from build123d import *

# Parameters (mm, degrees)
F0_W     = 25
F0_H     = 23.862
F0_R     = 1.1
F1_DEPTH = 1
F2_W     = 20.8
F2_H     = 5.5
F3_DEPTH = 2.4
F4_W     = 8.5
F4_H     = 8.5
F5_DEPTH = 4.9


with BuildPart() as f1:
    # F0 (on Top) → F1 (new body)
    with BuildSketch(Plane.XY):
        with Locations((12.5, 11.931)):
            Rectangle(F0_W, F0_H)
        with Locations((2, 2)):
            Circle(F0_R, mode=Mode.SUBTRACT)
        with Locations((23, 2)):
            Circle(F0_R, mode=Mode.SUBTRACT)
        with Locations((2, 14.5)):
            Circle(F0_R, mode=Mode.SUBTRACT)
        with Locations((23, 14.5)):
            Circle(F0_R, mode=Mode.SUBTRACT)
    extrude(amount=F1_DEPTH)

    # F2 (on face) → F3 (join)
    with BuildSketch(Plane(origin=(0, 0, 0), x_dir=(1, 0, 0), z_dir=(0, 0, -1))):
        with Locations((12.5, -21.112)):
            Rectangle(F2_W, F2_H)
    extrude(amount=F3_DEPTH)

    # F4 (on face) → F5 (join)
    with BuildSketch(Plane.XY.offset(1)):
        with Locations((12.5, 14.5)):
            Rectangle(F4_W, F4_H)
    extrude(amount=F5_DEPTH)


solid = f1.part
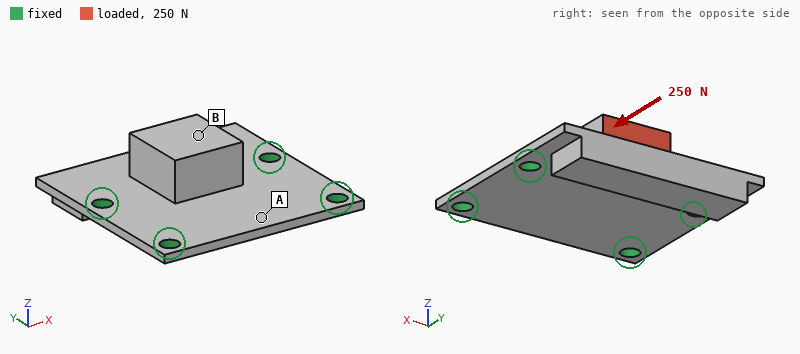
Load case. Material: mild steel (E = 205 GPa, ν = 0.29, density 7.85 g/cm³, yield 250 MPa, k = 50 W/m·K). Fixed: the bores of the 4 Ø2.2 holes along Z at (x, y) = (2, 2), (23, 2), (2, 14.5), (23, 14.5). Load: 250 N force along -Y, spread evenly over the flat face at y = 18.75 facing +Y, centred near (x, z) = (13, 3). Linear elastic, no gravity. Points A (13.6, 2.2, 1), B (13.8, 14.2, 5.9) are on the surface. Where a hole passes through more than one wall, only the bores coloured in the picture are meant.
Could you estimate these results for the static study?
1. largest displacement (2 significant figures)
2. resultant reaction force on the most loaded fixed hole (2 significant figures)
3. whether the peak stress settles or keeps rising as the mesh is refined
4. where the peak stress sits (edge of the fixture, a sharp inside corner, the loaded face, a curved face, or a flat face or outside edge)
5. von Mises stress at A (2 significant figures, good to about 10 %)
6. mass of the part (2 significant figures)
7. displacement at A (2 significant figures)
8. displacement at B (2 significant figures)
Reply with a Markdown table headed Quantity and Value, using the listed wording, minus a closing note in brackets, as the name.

| Quantity | Value |
|---|---|
| largest displacement | 17 µm |
| resultant reaction force on the most loaded fixed hole | 92 N |
| whether the peak stress settles or keeps rising as the mesh is refined | keeps rising |
| where the peak stress sits | edge of the fixture |
| von Mises stress at A | 23 MPa |
| mass of the part | 9.5 g |
| displacement at A | 6.6 µm |
| displacement at B | 10 µm |
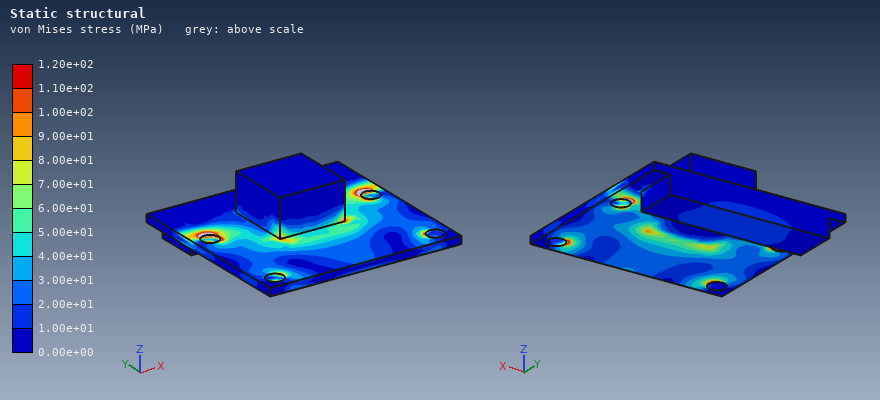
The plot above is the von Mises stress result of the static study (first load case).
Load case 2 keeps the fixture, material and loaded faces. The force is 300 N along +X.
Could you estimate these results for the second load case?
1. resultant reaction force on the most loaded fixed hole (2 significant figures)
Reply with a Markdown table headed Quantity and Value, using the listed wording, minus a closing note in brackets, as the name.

| Quantity | Value |
|---|---|
| resultant reaction force on the most loaded fixed hole | 150 N |
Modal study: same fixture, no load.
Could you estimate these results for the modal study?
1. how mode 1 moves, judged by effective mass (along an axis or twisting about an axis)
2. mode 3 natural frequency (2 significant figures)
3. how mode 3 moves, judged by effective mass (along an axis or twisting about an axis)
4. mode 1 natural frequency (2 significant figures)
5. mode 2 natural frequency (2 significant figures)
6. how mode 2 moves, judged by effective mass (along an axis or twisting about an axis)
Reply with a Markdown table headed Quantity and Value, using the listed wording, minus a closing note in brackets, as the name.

| Quantity | Value |
|---|---|
| how mode 1 moves, judged by effective mass | along Z |
| mode 3 natural frequency | 18 kHz |
| how mode 3 moves, judged by effective mass | twisting about Y |
| mode 1 natural frequency | 6200 Hz |
| mode 2 natural frequency | 11 kHz |
| how mode 2 moves, judged by effective mass | along Z |
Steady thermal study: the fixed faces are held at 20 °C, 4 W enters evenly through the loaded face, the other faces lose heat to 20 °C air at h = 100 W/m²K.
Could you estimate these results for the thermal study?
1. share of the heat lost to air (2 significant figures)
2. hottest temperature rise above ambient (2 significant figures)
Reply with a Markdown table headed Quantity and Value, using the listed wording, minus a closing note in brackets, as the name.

| Quantity | Value |
|---|---|
| share of the heat lost to air | 31 % |
| hottest temperature rise above ambient | 22 K |
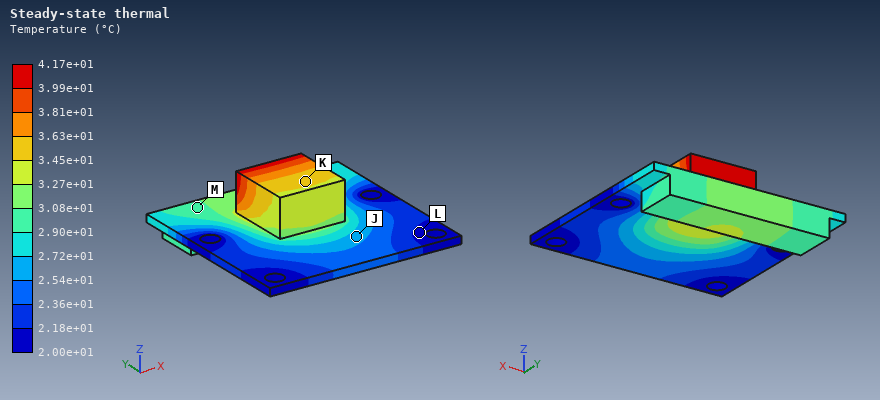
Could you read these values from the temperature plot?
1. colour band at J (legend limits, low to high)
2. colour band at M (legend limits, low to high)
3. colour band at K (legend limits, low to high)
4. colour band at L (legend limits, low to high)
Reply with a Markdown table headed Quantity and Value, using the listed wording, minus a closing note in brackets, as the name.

| Quantity | Value |
|---|---|
| colour band at J | 2.54e+01 to 2.72e+01 °C |
| colour band at M | 2.90e+01 to 3.08e+01 °C |
| colour band at K | 3.45e+01 to 3.63e+01 °C |
| colour band at L | 2.00e+01 to 2.18e+01 °C |
